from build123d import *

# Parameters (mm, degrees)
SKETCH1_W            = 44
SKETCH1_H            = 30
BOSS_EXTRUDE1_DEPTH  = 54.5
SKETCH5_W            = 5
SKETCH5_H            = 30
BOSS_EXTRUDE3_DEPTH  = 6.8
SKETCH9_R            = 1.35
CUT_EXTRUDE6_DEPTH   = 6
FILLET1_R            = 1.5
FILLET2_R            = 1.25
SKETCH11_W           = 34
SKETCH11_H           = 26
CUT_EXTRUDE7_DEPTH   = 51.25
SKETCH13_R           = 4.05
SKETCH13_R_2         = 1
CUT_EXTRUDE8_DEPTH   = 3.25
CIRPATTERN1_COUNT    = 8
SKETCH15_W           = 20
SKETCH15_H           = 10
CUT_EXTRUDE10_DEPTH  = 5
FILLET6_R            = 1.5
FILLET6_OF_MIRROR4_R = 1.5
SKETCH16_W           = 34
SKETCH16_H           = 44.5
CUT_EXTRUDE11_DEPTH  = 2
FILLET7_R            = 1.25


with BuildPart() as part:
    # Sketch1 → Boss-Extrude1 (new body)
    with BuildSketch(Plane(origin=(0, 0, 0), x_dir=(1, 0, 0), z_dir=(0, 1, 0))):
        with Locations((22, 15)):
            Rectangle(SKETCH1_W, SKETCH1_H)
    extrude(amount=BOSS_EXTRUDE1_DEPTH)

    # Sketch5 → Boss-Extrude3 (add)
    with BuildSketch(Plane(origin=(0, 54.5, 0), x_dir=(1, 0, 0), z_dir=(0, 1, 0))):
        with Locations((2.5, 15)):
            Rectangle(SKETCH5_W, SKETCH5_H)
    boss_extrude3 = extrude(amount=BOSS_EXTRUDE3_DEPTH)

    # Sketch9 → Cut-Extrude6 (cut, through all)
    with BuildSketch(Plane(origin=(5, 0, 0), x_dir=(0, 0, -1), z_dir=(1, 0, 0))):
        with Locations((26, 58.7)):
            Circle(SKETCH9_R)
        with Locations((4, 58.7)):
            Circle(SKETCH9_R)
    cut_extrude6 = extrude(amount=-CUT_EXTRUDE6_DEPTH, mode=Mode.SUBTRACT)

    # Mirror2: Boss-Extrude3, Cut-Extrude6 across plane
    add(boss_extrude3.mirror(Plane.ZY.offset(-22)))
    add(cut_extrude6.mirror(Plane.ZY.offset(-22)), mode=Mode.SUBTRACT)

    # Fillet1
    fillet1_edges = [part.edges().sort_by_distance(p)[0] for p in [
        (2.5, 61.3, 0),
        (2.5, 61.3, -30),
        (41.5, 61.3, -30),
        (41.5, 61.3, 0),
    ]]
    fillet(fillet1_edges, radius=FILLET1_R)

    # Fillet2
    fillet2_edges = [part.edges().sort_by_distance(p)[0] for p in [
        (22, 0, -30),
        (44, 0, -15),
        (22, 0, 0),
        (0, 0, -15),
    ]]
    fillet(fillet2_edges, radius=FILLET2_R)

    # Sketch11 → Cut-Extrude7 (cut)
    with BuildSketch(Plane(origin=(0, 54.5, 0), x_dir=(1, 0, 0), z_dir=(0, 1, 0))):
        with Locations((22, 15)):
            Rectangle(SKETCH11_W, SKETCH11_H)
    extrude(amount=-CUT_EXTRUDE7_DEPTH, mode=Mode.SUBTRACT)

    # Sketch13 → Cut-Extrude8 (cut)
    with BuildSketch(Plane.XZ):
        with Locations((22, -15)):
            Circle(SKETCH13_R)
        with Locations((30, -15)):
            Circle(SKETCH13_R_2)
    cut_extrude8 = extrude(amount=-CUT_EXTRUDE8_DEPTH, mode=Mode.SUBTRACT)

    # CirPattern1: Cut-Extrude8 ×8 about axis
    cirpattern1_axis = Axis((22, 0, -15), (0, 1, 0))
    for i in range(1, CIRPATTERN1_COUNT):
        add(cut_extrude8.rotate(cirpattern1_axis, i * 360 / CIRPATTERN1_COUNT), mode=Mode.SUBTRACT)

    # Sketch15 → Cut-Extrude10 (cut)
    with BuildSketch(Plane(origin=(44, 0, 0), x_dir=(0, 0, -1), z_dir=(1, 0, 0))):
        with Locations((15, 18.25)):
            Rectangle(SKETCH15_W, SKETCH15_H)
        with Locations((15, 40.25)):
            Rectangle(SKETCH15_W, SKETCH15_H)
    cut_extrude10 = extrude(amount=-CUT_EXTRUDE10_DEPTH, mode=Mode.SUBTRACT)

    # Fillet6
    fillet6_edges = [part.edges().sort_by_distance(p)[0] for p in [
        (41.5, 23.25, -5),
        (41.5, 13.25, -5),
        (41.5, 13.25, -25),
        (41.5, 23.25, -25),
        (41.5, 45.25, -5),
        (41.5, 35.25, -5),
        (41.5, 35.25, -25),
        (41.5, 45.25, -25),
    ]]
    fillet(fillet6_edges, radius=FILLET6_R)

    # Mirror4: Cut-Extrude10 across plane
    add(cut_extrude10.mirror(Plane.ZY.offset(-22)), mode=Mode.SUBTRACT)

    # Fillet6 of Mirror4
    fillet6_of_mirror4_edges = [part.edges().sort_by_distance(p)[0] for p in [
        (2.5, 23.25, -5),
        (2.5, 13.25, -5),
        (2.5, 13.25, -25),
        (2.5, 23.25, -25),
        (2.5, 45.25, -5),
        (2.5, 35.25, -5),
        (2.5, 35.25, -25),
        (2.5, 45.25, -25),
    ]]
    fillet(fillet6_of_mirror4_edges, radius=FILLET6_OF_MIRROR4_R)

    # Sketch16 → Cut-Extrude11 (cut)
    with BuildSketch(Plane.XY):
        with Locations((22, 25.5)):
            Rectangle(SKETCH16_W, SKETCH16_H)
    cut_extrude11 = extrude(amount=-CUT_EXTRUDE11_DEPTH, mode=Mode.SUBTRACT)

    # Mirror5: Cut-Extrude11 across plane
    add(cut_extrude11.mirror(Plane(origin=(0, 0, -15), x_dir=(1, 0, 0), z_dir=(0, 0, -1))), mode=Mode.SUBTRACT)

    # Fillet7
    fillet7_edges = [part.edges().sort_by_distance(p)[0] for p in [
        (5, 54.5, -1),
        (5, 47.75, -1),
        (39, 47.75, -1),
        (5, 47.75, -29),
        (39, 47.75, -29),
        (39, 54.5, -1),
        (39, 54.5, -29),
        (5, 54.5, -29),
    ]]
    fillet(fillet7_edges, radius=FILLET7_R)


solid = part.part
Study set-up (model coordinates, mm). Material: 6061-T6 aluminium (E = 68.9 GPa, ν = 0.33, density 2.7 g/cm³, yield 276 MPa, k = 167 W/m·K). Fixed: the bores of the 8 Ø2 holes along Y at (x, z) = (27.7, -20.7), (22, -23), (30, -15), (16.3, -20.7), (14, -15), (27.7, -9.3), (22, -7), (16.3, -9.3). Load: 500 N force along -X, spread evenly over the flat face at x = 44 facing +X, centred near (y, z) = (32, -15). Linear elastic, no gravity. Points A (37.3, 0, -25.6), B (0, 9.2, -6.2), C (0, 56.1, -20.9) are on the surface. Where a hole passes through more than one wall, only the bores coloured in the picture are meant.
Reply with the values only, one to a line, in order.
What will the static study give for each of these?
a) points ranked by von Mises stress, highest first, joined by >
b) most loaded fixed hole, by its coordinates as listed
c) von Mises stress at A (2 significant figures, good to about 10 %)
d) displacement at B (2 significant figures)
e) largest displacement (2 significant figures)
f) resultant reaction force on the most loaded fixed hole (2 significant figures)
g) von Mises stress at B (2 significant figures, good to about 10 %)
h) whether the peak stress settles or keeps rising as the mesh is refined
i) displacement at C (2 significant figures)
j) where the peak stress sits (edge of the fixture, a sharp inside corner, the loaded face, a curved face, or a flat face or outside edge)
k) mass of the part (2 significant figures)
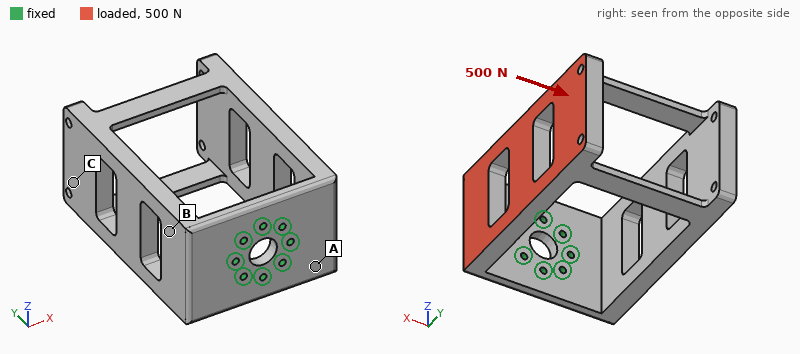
A > B > C
(30, -15)
84 MPa
0.12 mm
0.63 mm
420 N
30 MPa
keeps rising
0.59 mm
edge of the fixture
49 g
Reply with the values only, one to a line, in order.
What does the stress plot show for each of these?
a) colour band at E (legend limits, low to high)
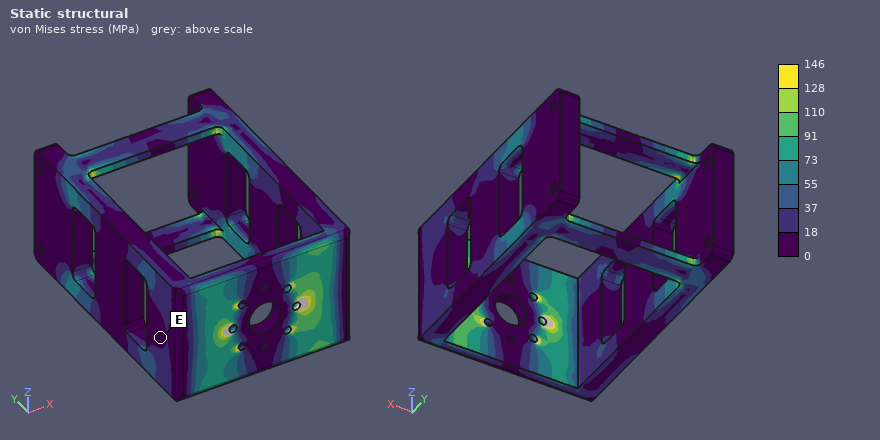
0 to 18 MPa
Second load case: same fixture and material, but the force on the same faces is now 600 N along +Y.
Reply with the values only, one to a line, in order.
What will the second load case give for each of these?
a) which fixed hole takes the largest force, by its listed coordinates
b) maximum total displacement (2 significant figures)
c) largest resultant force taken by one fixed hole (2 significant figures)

(30, -15)
0.24 mm
530 N
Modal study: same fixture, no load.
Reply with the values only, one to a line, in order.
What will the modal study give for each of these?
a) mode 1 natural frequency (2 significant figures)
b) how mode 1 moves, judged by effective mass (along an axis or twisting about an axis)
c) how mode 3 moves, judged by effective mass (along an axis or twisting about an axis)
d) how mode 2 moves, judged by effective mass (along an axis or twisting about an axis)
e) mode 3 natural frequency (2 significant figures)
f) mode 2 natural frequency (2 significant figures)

790 Hz
along X
twisting about Y
along Z
1600 Hz
1100 Hz
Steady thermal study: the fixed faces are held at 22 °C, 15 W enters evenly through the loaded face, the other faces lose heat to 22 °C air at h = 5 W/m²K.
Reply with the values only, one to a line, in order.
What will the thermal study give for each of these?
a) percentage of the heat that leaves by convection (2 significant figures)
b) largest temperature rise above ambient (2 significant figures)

4.6 %
35 K
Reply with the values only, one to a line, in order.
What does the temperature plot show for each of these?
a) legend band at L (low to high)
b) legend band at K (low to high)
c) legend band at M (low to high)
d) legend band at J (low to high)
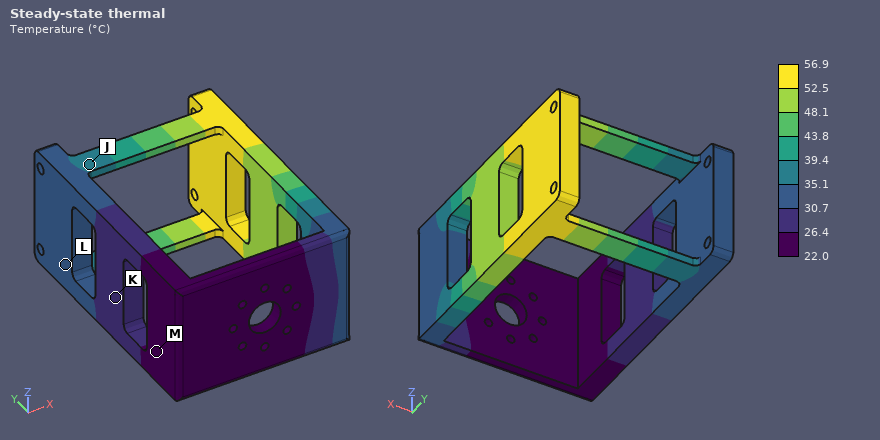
30.7 to 35.1 °C
26.4 to 30.7 °C
22.0 to 26.4 °C
35.1 to 39.4 °C
